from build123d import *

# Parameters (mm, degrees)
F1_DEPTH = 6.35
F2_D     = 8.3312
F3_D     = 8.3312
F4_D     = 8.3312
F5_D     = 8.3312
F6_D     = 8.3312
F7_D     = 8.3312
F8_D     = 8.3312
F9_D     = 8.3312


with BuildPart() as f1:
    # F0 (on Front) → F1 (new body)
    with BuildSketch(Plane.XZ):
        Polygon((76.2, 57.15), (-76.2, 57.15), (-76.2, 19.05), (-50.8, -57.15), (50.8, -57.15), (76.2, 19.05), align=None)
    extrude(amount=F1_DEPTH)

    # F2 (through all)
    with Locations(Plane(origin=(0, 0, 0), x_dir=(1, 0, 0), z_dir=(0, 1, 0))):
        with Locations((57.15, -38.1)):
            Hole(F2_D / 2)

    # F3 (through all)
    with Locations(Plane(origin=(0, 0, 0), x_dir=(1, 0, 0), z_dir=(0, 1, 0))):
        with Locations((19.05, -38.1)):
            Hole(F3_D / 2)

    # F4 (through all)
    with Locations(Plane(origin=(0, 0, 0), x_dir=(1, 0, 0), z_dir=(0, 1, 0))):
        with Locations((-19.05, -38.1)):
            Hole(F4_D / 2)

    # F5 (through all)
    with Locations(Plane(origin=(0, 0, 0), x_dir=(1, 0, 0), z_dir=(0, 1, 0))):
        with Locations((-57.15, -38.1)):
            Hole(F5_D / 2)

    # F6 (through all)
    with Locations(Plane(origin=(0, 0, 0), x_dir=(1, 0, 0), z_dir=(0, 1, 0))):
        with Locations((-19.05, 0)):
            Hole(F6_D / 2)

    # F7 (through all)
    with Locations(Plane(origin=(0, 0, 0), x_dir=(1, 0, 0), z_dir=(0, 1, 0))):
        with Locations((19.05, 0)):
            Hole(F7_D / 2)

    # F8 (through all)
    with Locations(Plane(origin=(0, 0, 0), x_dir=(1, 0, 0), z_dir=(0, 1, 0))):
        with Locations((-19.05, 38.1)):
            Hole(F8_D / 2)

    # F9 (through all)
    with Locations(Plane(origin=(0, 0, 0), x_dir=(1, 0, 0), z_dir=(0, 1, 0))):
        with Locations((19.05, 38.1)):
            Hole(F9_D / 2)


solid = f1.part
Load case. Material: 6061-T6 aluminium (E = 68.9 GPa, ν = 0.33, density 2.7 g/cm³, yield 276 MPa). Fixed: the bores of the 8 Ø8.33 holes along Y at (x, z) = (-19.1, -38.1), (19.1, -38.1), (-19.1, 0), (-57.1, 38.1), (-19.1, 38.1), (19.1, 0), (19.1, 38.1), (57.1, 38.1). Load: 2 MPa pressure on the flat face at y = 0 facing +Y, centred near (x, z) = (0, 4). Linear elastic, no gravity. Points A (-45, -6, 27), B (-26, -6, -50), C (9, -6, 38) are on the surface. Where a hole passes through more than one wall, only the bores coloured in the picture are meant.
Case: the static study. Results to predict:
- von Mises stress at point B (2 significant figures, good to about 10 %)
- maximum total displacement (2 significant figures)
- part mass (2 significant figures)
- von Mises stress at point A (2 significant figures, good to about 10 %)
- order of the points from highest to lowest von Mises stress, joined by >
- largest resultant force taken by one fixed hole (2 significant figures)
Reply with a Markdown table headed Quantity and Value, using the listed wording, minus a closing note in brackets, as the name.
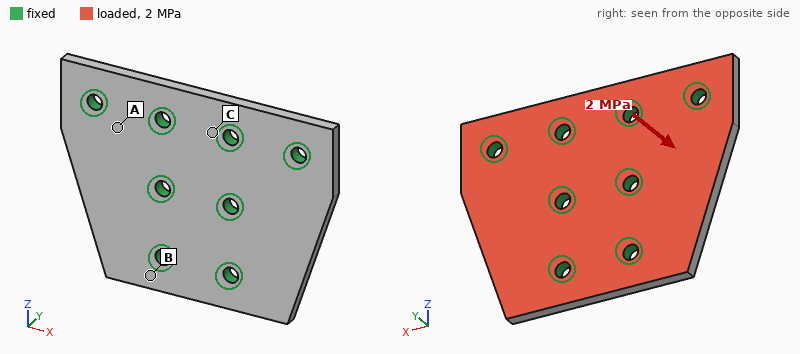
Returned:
| Quantity | Value |
|---|---|
| von Mises stress at point B | 96 MPa |
| maximum total displacement | 0.34 mm |
| part mass | 260 g |
| von Mises stress at point A | 59 MPa |
| order of the points from highest to lowest von Mises stress, joined by > | B > A > C |
| largest resultant force taken by one fixed hole | 4.5 kN |
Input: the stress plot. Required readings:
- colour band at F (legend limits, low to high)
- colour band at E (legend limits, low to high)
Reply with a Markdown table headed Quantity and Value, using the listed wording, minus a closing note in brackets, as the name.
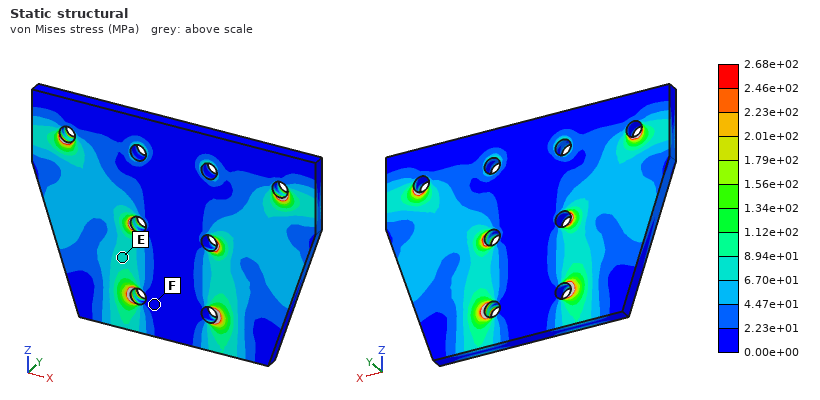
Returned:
| Quantity | Value |
|---|---|
| colour band at F | 0.00e+00 to 2.23e+01 MPa |
| colour band at E | 6.70e+01 to 8.94e+01 MPa |
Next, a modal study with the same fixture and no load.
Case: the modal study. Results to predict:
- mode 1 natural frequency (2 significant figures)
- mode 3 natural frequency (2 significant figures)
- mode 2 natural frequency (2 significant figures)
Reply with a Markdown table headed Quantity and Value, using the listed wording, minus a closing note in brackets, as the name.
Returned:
| Quantity | Value |
|---|---|
| mode 1 natural frequency | 3900 Hz |
| mode 3 natural frequency | 6700 Hz |
| mode 2 natural frequency | 3900 Hz |
